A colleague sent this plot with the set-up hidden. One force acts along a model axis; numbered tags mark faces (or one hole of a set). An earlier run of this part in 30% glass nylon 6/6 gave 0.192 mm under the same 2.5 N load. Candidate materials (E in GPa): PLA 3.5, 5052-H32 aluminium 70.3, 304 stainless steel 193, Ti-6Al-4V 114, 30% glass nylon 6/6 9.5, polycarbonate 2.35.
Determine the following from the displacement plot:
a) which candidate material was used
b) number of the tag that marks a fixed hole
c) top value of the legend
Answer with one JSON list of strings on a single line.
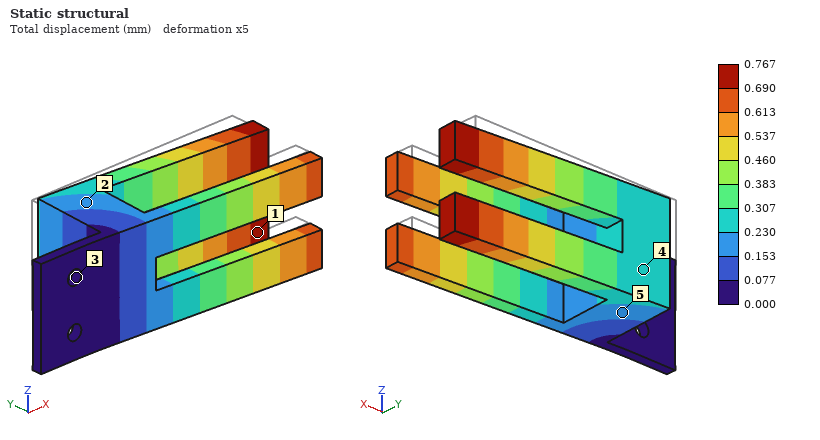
["polycarbonate", "3", "0.767 mm"]
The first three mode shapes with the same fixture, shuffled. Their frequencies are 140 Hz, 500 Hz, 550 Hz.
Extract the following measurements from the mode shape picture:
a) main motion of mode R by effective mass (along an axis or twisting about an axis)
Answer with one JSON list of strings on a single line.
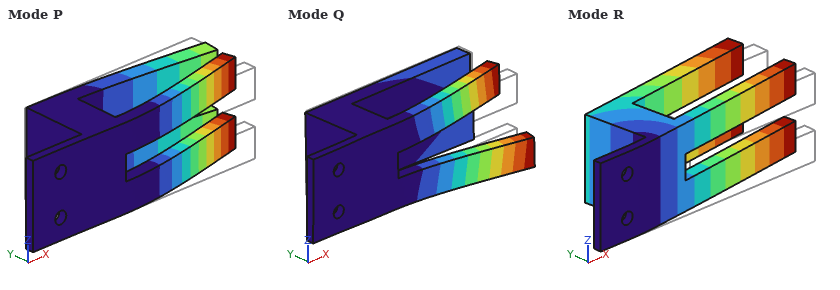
["along Y"]
